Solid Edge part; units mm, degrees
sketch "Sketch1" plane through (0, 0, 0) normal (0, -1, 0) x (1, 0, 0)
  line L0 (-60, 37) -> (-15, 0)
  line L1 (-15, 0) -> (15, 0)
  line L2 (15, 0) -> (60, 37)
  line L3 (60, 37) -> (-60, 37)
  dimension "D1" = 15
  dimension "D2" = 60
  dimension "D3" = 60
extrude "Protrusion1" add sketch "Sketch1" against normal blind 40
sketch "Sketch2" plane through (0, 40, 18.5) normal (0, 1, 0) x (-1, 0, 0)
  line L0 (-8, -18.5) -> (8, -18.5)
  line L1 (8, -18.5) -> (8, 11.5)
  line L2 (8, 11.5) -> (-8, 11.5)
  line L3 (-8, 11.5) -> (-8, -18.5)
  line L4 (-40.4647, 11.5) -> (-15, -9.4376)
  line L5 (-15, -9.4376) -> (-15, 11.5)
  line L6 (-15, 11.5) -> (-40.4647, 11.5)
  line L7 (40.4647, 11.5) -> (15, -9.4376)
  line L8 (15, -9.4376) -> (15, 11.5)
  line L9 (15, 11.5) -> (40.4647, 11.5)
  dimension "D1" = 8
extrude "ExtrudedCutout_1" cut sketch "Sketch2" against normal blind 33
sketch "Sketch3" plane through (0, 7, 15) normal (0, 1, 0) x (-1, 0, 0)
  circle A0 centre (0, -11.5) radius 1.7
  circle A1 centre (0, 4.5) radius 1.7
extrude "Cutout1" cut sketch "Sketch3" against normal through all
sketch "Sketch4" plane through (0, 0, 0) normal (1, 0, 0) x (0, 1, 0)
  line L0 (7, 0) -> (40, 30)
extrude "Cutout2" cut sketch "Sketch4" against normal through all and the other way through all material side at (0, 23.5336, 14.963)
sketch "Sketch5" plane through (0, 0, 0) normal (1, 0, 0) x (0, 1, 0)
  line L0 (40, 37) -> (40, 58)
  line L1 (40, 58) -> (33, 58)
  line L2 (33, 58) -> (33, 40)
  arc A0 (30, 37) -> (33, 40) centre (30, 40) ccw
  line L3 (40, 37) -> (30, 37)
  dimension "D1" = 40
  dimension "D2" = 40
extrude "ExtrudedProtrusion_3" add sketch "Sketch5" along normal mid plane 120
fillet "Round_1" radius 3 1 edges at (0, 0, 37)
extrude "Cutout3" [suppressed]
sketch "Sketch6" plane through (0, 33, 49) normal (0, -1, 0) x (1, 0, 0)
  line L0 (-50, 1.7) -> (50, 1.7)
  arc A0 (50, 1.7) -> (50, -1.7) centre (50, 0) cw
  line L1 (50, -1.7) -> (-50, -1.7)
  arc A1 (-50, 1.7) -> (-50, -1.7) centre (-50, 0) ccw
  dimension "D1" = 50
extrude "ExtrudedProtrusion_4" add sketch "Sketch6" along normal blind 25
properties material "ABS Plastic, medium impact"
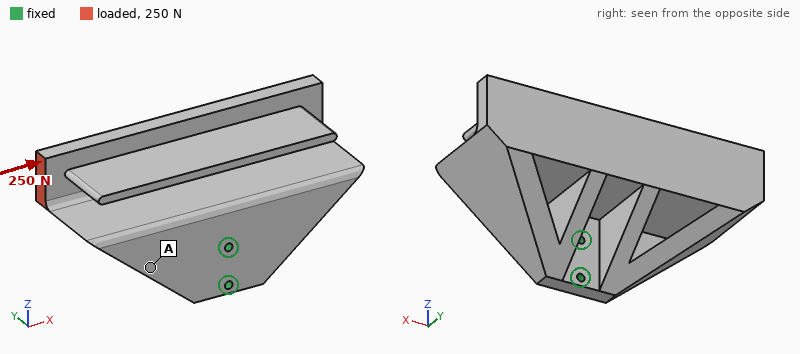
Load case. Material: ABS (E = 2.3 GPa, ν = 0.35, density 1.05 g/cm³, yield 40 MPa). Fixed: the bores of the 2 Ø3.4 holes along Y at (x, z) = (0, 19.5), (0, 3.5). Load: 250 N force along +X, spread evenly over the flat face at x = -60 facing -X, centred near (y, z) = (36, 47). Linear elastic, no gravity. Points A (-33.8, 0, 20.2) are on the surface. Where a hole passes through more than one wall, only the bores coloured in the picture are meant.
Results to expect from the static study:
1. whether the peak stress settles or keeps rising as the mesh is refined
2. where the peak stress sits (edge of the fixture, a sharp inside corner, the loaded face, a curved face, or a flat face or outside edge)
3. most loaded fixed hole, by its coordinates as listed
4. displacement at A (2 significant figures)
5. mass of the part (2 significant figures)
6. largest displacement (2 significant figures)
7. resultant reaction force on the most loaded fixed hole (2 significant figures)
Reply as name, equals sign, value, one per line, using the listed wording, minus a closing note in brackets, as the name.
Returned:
whether the peak stress settles or keeps rising as the mesh is refined = keeps rising
where the peak stress sits = edge of the fixture
most loaded fixed hole, by its coordinates as listed = (0, 19.5)
displacement at A = 0.64 mm
mass of the part = 93 g
largest displacement = 1.5 mm
resultant reaction force on the most loaded fixed hole = 620 N
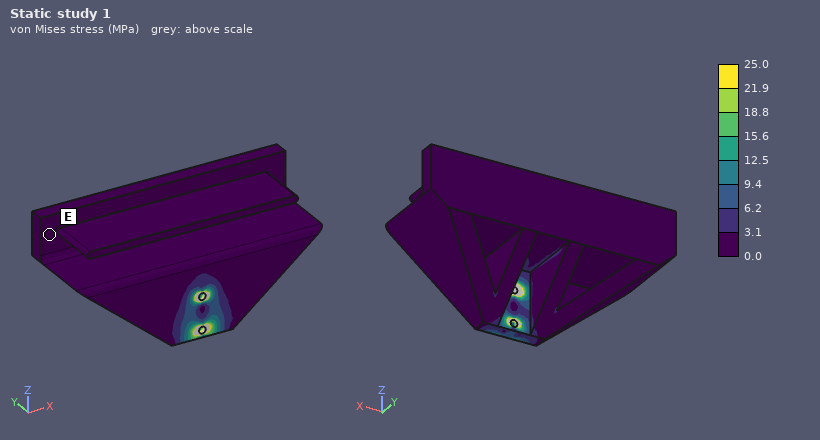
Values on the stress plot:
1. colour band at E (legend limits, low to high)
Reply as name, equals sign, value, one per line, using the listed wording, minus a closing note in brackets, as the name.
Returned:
colour band at E = 0.0 to 3.1 MPa
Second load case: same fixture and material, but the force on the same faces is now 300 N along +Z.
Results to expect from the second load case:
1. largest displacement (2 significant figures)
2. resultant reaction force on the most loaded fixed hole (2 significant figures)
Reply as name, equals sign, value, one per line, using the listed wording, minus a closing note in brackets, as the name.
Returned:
largest displacement = 1.5 mm
resultant reaction force on the most loaded fixed hole = 1.1 kN
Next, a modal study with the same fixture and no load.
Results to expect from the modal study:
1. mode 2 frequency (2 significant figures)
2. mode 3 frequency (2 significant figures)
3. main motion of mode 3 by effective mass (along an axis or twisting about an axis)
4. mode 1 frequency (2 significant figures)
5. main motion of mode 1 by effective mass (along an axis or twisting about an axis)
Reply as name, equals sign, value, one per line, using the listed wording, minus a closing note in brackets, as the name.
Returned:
mode 2 frequency = 520 Hz
mode 3 frequency = 690 Hz
main motion of mode 3 by effective mass = along X
mode 1 frequency = 280 Hz
main motion of mode 1 by effective mass = along X
